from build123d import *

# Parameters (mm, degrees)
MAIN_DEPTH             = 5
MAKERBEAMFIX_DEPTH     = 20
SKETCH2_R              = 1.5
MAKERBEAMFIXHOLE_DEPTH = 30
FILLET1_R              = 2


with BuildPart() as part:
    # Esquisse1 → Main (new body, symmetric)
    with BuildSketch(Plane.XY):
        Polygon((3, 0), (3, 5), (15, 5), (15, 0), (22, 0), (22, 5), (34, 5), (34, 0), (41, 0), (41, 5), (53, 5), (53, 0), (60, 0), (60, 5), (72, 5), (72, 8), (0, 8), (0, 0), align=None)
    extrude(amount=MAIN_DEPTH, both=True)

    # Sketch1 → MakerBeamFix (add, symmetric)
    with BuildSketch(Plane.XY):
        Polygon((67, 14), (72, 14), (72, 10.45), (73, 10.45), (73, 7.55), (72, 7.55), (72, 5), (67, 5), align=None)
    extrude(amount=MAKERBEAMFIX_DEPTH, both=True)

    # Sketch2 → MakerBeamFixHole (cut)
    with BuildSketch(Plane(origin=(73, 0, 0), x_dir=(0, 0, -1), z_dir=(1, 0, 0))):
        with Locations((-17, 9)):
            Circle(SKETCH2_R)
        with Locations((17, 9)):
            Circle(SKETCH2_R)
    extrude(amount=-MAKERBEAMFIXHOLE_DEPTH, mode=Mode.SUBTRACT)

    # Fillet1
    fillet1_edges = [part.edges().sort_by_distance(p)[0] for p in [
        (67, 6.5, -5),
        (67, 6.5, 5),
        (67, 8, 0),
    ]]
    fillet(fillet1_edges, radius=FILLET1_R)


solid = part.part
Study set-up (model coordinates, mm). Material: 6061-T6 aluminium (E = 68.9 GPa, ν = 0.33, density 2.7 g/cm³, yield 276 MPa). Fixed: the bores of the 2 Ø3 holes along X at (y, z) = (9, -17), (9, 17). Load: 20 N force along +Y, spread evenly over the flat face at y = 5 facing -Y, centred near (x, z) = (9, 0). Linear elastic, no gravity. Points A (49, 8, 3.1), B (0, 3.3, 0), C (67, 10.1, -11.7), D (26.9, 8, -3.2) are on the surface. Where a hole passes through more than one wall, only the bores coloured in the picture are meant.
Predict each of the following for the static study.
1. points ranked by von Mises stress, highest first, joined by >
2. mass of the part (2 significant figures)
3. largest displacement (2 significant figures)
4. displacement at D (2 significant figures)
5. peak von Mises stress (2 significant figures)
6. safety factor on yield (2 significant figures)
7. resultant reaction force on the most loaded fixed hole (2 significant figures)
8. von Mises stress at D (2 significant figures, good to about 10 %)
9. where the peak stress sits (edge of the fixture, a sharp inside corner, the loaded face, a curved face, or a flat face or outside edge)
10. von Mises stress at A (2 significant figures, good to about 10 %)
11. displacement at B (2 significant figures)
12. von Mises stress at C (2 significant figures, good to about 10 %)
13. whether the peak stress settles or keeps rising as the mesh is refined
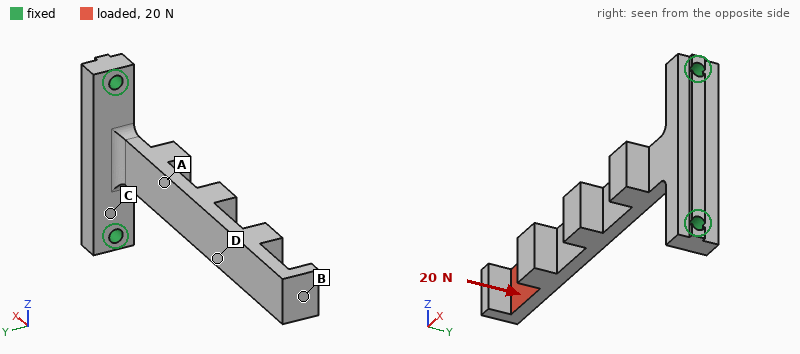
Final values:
A > D > C > B
14 g
0.91 mm
0.42 mm
100 MPa
2.7
14 N
24 MPa
a curved face
53 MPa
0.90 mm
16 MPa
settles
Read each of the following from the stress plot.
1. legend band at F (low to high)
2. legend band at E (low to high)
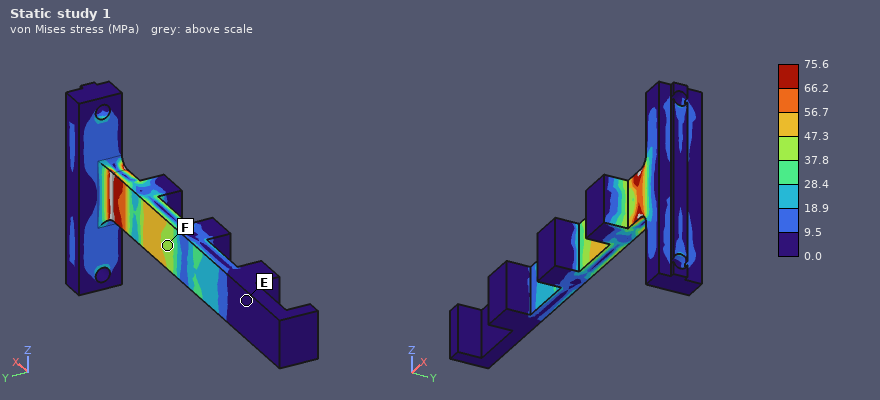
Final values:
37.8 to 47.3 MPa
0.0 to 9.5 MPa
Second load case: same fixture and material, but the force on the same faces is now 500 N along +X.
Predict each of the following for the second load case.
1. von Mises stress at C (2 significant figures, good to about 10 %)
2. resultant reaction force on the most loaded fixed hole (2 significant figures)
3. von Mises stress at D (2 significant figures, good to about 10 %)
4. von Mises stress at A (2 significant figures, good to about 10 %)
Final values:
28 MPa
260 N
33 MPa
33 MPa
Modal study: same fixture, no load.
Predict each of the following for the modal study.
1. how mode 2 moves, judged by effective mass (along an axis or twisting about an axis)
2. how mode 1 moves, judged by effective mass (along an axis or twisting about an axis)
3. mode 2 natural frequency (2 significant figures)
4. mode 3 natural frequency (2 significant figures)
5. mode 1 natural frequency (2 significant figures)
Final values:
along Z
along Y
1300 Hz
2700 Hz
450 Hz
